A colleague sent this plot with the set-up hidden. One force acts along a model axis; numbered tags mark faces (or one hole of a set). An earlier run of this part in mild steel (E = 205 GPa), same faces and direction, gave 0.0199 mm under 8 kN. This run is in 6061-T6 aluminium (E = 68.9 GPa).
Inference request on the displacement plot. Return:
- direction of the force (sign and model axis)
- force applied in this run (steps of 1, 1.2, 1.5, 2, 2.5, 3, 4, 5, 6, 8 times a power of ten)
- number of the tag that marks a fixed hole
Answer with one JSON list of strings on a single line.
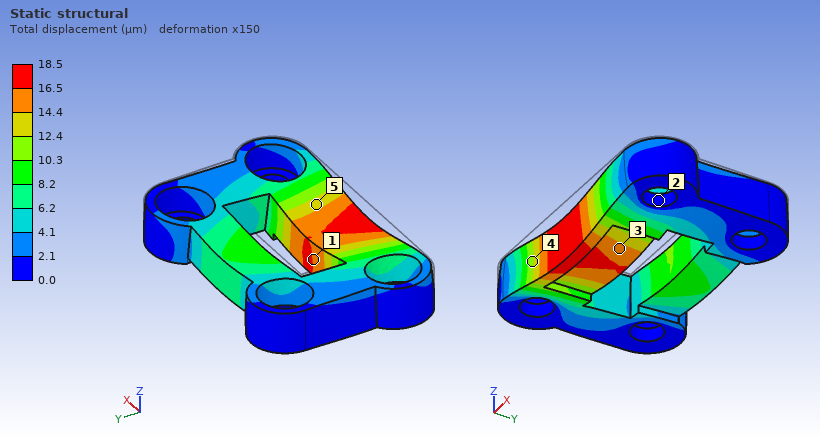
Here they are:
["-Z", "2.5 kN", "2"]
